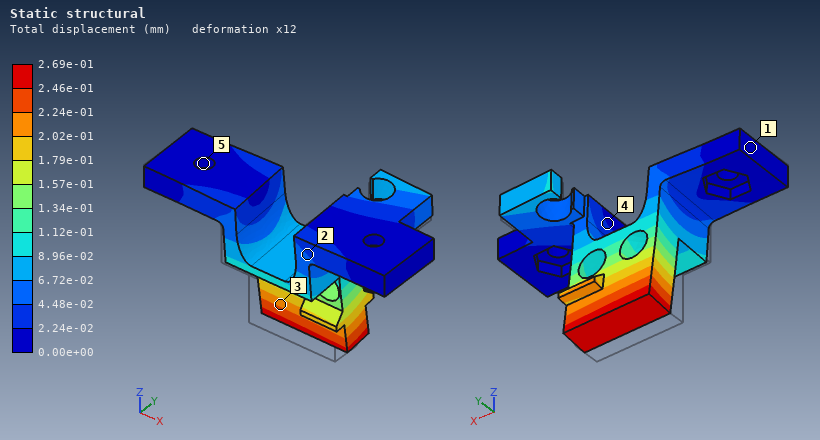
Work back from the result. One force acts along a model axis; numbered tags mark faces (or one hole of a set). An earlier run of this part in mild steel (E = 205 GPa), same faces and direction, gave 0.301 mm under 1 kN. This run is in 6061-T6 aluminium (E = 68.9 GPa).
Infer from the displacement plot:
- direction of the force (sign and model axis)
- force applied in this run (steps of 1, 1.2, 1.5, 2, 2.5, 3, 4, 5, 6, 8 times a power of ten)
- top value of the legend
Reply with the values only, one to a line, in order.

+Y
300 N
2.69e-01 mm
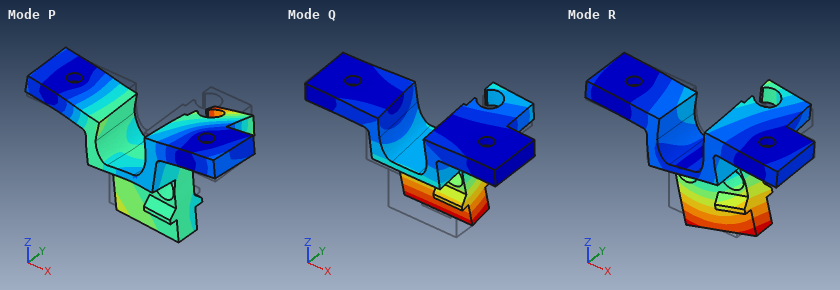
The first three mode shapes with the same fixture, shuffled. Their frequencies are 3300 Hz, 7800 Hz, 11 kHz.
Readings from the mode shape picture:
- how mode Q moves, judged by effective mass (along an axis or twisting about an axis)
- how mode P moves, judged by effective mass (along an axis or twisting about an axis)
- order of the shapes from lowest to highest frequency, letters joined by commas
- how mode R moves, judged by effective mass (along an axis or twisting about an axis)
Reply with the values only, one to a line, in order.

along Y
along Z
Q, R, P
along X
